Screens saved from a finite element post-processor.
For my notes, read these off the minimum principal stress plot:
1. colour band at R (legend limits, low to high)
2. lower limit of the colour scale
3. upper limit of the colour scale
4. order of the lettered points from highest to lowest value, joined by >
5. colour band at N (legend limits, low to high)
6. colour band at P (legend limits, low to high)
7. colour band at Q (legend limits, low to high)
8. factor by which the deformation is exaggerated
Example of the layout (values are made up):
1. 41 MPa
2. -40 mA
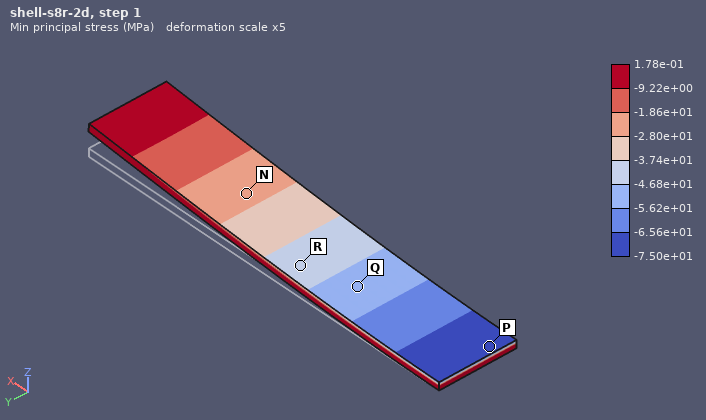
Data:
1. -4.68e+01 to -3.74e+01 MPa
2. -7.50e+01 MPa
3. 1.78e-01 MPa
4. N > R > Q > P
5. -2.80e+01 to -1.86e+01 MPa
6. -7.50e+01 to -6.56e+01 MPa
7. -5.62e+01 to -4.68e+01 MPa
8. 5
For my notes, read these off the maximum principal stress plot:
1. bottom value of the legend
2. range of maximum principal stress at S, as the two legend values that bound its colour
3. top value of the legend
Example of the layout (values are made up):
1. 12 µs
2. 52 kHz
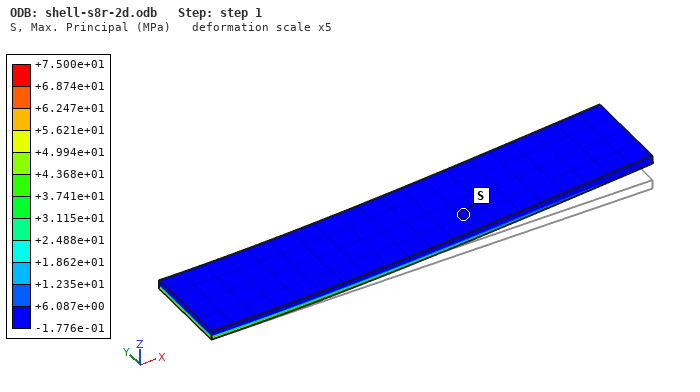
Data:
1. -1.776e-01 MPa
2. -1.776e-01 to +6.087e+00 MPa
3. +7.500e+01 MPa
